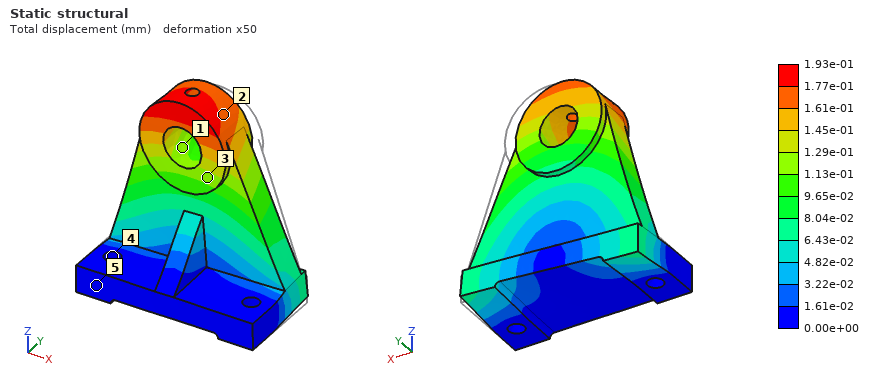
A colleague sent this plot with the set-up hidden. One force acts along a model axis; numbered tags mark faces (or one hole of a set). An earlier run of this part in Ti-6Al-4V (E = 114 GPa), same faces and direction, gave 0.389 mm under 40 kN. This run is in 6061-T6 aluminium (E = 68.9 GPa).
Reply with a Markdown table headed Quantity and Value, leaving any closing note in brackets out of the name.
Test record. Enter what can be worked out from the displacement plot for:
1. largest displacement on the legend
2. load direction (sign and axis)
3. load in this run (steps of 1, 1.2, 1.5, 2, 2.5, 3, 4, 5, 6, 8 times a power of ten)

| Quantity | Value |
|---|---|
| largest displacement on the legend | 1.93e-01 mm |
| load direction | -X |
| load in this run | 12 kN |
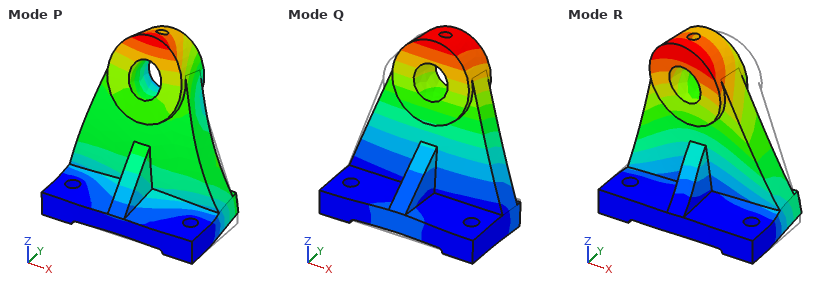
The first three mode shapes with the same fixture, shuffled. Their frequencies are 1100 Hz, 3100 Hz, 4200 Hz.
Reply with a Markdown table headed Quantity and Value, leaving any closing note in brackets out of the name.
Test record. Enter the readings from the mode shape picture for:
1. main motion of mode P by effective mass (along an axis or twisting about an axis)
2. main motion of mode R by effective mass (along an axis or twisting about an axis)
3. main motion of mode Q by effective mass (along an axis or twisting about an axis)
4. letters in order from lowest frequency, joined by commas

| Quantity | Value |
|---|---|
| main motion of mode P by effective mass | along Z |
| main motion of mode R by effective mass | along X |
| main motion of mode Q by effective mass | along Y |
| letters in order from lowest frequency, joined by commas | Q, R, P |
